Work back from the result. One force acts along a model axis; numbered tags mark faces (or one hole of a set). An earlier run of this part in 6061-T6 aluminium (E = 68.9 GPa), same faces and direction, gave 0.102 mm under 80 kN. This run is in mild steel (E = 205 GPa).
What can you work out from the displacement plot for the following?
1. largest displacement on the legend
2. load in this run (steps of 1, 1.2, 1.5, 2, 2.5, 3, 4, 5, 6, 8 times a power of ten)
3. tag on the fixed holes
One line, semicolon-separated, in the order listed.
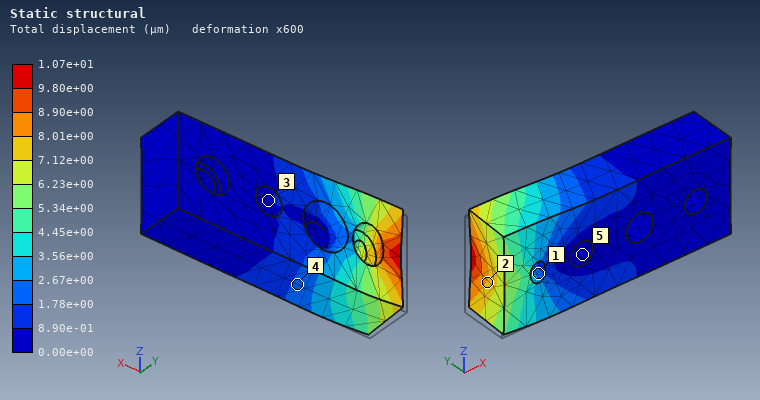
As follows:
1.07e+01 µm; 25 kN; 5
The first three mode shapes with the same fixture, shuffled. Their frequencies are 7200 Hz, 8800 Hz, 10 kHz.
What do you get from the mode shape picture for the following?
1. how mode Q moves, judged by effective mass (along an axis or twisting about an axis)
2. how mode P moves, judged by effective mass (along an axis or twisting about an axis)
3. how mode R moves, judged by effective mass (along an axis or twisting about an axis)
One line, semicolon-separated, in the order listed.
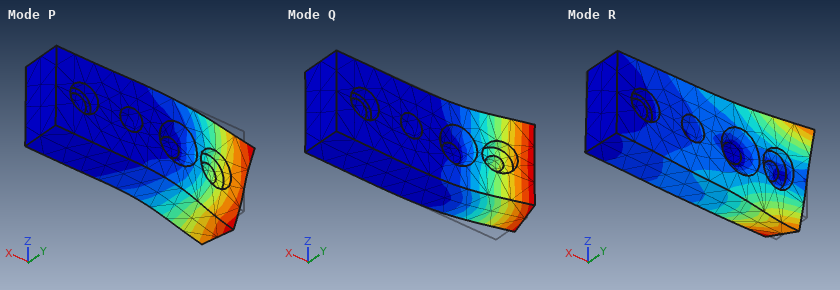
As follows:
along Y; along Z; twisting about X
